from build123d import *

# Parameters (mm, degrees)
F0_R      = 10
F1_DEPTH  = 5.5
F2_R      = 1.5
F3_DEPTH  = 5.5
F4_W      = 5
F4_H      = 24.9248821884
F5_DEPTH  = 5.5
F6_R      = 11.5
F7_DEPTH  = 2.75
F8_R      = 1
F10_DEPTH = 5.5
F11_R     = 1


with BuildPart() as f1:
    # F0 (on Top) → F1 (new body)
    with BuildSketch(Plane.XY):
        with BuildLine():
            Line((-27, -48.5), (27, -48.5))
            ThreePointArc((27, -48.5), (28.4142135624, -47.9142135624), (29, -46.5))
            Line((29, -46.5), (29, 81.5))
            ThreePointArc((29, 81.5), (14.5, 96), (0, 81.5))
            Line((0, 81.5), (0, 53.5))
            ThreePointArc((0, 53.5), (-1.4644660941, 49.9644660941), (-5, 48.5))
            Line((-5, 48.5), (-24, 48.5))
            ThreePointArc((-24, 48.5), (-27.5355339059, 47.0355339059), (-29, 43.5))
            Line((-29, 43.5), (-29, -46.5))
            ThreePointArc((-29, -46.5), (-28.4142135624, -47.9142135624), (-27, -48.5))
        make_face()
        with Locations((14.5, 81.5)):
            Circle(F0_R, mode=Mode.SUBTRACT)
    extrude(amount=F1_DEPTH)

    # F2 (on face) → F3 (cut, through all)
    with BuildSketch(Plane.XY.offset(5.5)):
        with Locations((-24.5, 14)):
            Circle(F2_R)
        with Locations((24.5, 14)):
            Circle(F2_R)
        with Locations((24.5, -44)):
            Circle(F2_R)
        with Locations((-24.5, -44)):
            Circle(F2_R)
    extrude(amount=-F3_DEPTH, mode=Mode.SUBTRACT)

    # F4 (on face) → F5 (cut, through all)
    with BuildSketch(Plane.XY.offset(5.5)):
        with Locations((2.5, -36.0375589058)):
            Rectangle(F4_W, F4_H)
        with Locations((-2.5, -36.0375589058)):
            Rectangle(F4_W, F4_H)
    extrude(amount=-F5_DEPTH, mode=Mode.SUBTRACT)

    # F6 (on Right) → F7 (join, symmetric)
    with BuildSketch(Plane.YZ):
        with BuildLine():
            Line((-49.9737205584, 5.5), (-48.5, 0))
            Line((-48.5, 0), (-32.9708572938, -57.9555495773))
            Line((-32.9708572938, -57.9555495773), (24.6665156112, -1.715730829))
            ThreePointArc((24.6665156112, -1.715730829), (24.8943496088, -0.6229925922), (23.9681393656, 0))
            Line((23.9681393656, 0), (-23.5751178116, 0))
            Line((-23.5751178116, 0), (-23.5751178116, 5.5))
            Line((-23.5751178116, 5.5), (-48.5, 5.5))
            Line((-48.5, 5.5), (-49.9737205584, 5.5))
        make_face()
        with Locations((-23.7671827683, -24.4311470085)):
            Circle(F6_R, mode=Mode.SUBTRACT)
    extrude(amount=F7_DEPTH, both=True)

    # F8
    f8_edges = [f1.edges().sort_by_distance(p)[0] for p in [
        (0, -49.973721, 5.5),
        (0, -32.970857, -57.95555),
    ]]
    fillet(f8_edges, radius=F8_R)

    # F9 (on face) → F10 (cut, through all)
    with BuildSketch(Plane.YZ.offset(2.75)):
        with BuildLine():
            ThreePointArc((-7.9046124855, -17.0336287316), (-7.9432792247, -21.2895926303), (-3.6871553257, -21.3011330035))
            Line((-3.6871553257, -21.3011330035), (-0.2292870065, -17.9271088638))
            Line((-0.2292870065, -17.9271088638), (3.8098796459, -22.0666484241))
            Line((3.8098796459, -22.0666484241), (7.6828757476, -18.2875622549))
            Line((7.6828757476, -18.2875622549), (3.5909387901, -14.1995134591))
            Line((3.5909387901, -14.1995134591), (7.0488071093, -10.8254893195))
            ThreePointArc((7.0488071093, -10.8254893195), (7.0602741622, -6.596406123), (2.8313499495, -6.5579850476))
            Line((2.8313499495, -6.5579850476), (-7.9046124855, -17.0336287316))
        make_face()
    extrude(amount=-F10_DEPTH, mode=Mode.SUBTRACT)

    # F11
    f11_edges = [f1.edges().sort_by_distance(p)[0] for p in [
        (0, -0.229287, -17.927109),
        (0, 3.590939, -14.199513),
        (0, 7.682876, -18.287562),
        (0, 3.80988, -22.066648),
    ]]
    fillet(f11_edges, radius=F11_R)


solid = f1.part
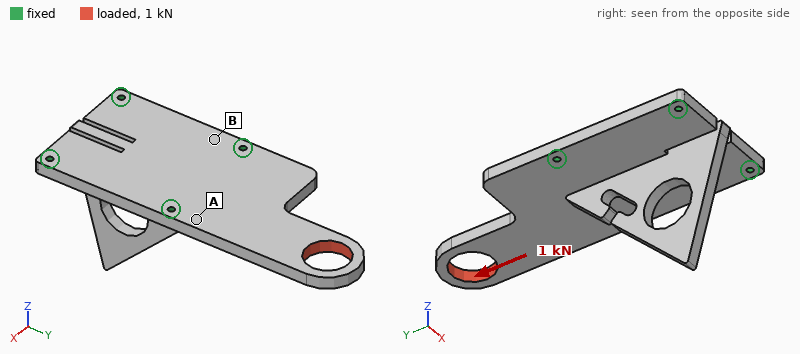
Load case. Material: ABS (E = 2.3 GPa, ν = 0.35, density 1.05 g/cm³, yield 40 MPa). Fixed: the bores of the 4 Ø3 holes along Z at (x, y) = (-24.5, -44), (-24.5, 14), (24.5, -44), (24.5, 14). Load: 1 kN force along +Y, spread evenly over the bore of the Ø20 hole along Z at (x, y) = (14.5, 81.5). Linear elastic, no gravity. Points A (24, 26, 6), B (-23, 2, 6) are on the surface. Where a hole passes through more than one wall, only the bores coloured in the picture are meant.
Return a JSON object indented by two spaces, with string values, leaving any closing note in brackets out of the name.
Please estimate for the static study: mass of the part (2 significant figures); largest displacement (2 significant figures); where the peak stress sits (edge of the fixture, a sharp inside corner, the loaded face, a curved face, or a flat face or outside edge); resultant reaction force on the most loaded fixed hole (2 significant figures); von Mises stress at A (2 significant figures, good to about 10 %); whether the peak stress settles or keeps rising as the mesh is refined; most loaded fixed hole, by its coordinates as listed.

{
  "mass of the part": "47 g",
  "largest displacement": "0.49 mm",
  "where the peak stress sits": "a sharp inside corner",
  "resultant reaction force on the most loaded fixed hole": "690 N",
  "von Mises stress at A": "8.7 MPa",
  "whether the peak stress settles or keeps rising as the mesh is refined": "keeps rising",
  "most loaded fixed hole, by its coordinates as listed": "(24.5, 14)"
}
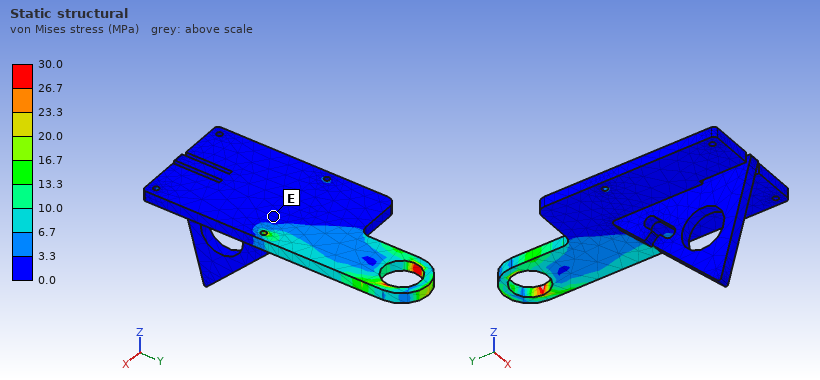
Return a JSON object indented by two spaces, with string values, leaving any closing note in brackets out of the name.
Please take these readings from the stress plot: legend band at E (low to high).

{
  "legend band at E": "0.0 to 3.3 MPa"
}
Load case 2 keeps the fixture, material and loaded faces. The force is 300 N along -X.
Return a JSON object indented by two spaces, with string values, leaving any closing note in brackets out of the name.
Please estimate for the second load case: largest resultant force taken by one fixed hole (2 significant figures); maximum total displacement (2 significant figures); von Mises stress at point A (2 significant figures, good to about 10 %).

{
  "largest resultant force taken by one fixed hole": "420 N",
  "maximum total displacement": "1.1 mm",
  "von Mises stress at point A": "6.7 MPa"
}
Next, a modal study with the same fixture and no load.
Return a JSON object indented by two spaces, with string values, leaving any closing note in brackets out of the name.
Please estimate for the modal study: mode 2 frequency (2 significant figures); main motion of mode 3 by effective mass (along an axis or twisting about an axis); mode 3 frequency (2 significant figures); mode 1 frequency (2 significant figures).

{
  "mode 2 frequency": "430 Hz",
  "main motion of mode 3 by effective mass": "along Z",
  "mode 3 frequency": "760 Hz",
  "mode 1 frequency": "310 Hz"
}
